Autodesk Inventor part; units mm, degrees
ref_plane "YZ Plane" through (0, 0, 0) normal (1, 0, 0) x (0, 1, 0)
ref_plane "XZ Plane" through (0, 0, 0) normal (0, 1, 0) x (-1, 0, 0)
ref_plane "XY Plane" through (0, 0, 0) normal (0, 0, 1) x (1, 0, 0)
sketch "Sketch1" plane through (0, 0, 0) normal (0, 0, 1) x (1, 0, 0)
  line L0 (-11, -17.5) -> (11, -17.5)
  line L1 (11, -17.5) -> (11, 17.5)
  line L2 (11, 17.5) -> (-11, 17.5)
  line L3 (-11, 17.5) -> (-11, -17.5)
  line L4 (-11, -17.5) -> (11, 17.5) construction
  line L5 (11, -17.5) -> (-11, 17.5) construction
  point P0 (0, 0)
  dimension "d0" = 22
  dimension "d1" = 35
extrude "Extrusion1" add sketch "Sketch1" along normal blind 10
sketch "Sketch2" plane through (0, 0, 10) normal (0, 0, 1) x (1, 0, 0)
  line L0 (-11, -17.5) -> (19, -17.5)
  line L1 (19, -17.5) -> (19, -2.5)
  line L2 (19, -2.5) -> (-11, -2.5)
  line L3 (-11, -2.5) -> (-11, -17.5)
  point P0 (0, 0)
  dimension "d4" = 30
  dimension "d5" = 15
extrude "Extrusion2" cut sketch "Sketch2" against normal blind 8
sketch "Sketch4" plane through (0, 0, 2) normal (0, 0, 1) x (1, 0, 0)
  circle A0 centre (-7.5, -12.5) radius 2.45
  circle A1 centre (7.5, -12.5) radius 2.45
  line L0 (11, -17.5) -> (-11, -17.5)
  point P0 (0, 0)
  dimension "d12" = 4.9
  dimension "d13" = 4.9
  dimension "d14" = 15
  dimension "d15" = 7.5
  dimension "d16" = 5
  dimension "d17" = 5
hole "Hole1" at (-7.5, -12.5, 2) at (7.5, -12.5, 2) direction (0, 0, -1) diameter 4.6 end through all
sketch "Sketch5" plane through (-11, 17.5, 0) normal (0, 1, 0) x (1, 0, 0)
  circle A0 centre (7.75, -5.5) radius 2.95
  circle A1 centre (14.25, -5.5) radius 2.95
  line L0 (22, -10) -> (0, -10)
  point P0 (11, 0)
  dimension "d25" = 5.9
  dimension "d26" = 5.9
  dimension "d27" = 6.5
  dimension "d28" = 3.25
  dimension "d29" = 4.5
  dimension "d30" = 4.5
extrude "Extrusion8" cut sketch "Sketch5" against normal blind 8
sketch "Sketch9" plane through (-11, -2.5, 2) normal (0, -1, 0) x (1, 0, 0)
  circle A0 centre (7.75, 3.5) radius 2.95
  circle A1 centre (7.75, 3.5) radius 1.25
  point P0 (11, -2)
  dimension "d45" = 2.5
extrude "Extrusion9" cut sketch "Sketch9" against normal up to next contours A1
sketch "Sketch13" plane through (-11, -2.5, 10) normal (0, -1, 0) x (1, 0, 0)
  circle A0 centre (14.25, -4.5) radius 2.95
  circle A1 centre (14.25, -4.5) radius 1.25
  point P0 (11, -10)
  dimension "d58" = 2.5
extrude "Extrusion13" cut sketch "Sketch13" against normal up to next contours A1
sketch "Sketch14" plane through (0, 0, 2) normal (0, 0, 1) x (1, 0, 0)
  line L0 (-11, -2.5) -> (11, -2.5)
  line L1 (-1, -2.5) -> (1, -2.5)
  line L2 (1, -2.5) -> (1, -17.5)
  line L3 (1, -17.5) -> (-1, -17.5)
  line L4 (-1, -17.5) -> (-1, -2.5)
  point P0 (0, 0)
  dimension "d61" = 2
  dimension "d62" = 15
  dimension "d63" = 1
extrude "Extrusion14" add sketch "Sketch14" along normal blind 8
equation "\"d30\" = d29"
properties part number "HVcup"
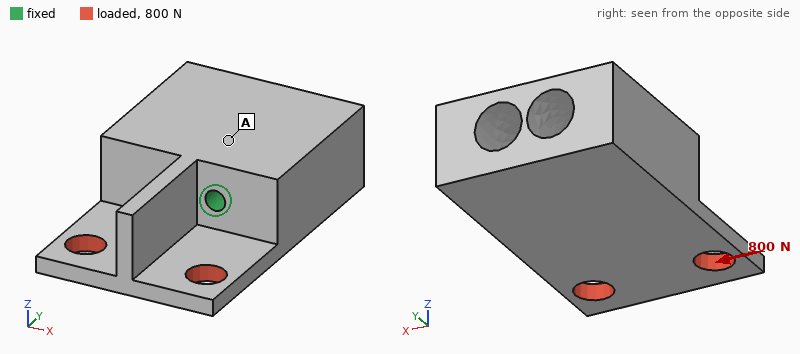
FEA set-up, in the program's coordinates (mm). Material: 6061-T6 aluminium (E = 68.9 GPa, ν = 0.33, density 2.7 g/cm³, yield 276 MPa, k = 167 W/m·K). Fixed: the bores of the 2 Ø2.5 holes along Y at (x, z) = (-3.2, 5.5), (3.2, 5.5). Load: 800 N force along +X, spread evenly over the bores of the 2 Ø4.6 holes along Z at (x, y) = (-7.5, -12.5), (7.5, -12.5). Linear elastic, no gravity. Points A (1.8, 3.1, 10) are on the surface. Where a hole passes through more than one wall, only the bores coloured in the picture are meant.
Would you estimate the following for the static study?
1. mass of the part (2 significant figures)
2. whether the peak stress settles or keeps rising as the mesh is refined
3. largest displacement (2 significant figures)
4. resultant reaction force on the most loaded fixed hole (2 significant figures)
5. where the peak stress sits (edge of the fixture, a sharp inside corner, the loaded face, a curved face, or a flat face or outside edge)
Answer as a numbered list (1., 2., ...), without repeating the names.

1. 13 g
2. keeps rising
3. 27 µm
4. 870 N
5. edge of the fixture
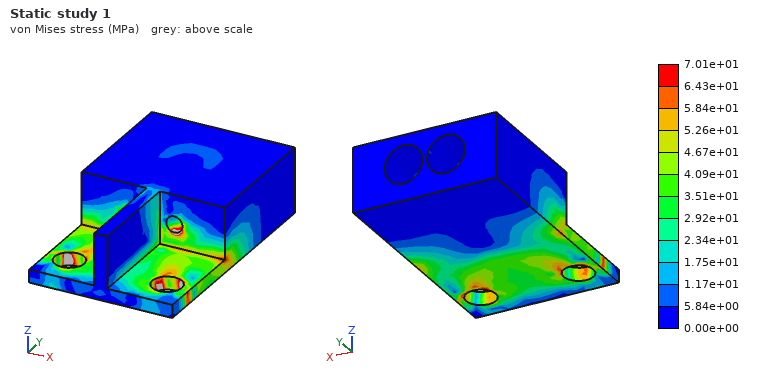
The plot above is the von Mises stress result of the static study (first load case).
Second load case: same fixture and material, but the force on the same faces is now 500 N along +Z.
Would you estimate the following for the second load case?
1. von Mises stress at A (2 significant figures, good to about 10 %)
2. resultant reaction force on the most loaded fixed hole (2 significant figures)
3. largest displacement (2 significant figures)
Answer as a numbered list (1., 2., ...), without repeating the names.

1. 11 MPa
2. 250 N
3. 0.11 mm
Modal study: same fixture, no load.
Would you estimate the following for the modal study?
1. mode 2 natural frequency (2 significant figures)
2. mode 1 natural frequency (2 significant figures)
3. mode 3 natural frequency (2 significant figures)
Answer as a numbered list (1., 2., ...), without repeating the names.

1. 15 kHz
2. 13 kHz
3. 23 kHz
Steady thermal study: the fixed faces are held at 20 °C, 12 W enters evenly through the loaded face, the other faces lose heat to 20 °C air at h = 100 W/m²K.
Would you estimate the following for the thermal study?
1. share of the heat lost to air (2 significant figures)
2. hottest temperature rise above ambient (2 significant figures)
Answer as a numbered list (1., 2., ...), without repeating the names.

1. 9.2 %
2. 22 K
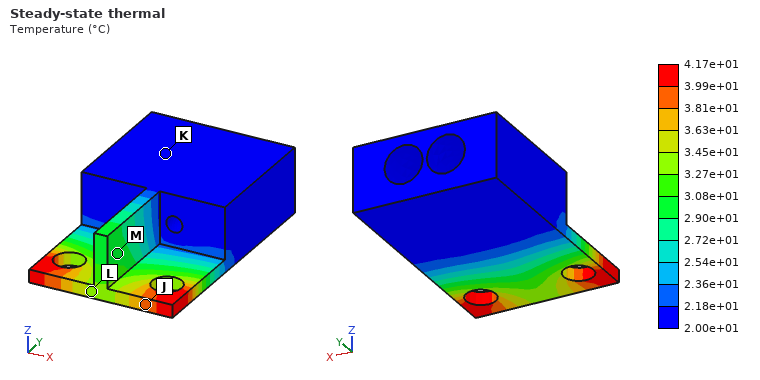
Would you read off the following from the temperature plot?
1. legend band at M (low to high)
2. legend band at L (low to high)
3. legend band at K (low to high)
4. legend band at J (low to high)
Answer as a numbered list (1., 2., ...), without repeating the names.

1. 2.90e+01 to 3.08e+01 °C
2. 3.27e+01 to 3.45e+01 °C
3. 2.00e+01 to 2.18e+01 °C
4. 3.81e+01 to 3.99e+01 °C
